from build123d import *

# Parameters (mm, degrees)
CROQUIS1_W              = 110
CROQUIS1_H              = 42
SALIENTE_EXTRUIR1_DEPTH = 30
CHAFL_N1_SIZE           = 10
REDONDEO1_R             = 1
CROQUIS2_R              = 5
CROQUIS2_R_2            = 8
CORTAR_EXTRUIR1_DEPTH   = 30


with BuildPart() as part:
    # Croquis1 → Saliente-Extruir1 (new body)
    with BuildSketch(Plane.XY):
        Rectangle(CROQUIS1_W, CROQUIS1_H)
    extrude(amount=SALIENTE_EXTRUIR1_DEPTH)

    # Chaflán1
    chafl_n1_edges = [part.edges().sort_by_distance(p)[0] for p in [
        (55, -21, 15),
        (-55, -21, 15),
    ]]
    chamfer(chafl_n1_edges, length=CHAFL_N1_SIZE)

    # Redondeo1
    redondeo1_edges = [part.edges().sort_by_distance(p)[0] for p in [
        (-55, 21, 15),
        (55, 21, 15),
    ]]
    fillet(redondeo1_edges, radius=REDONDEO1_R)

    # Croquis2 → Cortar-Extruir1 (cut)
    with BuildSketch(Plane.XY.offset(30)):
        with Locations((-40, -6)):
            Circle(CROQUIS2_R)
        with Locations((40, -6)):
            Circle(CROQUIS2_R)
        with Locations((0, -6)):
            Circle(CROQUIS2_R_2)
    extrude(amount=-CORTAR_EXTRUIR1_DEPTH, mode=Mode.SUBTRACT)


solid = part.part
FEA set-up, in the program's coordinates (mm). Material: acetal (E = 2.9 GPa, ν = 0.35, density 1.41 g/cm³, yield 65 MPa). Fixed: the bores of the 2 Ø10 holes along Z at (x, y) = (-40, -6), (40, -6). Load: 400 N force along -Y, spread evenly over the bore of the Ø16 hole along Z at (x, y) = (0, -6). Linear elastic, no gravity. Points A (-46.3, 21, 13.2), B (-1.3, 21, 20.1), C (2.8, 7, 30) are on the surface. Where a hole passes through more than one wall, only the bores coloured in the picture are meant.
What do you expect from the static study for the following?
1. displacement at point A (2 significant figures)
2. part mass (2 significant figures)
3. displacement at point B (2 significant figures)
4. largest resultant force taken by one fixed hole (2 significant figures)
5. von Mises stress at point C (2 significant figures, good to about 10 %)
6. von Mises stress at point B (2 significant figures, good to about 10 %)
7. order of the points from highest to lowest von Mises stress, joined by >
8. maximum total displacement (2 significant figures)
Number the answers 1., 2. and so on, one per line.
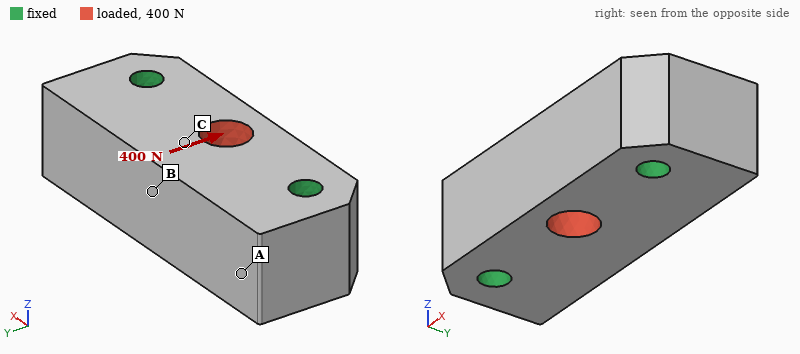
1. 3.8 µm
2. 180 g
3. 8.5 µm
4. 210 N
5. 0.33 MPa
6. 0.64 MPa
7. B > C > A
8. 13 µm
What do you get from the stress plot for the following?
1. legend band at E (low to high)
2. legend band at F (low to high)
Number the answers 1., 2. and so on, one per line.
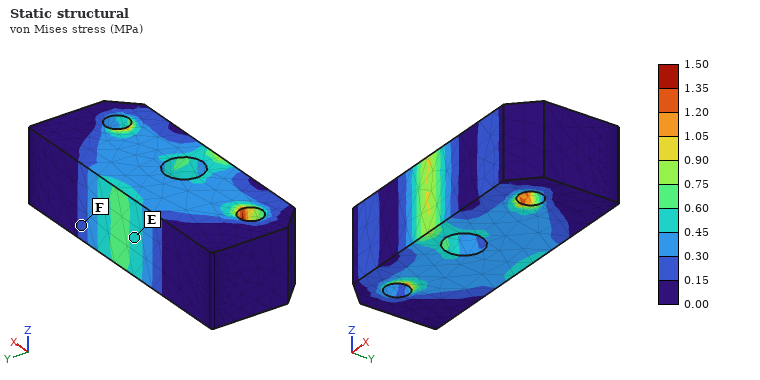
1. 0.45 to 0.60 MPa
2. 0.15 to 0.30 MPa
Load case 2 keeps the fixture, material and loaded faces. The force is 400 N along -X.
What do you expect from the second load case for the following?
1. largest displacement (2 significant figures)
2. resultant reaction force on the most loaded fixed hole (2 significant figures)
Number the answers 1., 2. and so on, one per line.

1. 3.3 µm
2. 200 N
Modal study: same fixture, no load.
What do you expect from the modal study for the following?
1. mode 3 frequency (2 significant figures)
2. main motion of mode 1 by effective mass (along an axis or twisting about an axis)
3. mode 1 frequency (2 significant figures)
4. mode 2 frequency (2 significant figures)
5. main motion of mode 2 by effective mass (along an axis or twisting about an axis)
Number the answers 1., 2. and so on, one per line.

1. 4800 Hz
2. along Z
3. 3500 Hz
4. 4000 Hz
5. along Y
